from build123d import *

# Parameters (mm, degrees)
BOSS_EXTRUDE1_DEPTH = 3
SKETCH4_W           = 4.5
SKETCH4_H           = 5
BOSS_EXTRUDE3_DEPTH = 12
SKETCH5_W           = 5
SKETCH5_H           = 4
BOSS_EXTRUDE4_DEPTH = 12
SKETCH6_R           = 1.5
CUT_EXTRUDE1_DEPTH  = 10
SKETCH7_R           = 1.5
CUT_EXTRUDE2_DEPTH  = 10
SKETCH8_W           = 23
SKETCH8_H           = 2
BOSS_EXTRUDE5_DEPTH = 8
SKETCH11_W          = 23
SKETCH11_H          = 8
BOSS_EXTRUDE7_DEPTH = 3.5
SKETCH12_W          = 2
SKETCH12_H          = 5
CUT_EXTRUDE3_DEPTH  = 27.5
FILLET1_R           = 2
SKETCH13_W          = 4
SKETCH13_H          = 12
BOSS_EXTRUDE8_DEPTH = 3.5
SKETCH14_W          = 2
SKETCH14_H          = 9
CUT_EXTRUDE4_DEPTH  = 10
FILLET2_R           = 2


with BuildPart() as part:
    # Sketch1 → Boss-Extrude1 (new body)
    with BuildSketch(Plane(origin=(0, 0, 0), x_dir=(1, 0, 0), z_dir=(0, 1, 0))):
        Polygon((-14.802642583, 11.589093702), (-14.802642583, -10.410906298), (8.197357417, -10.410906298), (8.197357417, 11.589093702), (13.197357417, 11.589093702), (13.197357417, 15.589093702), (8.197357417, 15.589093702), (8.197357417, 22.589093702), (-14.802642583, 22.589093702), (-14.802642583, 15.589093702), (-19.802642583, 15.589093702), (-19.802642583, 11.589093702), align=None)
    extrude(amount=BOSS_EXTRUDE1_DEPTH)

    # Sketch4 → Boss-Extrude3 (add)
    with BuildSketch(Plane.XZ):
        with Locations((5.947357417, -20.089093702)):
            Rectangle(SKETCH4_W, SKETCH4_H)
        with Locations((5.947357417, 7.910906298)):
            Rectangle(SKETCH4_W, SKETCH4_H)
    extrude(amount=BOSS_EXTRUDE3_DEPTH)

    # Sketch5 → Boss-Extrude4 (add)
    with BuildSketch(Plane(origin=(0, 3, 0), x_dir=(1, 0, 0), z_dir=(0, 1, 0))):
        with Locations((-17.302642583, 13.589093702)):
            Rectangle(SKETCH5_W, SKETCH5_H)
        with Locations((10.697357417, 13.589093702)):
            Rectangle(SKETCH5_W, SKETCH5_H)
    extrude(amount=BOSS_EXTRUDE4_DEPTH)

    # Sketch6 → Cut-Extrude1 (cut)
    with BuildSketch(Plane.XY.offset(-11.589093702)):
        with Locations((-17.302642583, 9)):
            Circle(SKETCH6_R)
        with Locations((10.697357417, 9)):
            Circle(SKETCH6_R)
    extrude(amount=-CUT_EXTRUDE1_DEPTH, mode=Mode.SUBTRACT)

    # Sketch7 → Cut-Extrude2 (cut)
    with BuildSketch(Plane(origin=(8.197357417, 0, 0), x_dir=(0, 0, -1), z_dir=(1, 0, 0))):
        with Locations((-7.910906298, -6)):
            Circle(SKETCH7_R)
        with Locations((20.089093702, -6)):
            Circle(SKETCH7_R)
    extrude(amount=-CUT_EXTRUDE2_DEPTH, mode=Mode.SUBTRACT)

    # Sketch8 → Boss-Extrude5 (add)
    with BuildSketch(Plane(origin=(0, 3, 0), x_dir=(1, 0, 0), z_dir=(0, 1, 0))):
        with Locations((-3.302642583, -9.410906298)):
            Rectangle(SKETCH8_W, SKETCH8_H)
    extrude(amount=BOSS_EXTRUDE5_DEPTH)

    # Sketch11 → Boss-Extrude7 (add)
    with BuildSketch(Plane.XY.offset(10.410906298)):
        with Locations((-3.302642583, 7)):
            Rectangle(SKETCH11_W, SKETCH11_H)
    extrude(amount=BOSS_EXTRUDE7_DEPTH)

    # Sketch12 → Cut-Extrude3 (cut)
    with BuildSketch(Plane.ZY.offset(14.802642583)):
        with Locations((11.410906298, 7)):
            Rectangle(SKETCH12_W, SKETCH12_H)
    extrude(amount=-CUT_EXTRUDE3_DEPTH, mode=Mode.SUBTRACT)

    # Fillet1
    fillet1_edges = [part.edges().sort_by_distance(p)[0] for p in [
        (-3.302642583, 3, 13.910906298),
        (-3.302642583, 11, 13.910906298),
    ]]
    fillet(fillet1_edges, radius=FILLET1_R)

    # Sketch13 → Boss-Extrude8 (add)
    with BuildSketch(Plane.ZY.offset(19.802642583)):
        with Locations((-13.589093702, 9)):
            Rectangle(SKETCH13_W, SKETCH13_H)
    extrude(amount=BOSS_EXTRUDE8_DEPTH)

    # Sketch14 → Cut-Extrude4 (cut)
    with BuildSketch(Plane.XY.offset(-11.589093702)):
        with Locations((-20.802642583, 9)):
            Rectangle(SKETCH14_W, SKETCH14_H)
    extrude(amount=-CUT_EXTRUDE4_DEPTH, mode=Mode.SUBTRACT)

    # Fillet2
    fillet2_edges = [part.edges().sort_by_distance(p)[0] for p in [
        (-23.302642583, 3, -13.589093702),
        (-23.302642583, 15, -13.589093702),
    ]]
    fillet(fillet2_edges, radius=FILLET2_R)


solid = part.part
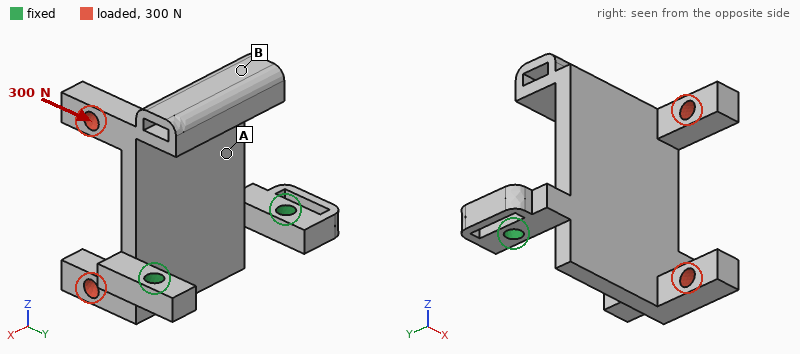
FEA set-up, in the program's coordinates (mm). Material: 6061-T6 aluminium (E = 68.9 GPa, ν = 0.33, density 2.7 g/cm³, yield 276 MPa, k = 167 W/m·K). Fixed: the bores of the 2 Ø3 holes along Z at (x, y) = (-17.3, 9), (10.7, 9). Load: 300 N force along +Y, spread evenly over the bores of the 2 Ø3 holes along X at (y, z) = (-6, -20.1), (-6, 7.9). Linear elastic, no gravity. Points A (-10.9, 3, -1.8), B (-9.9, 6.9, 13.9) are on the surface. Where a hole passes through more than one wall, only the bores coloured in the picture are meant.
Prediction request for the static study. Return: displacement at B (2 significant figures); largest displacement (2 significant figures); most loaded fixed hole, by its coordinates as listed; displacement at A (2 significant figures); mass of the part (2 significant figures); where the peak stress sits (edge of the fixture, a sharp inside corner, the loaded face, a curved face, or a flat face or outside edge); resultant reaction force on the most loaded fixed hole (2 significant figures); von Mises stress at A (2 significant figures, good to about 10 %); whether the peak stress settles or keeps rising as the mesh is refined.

0.38 mm
0.48 mm
(10.7, 9)
0.13 mm
11 g
a sharp inside corner
290 N
44 MPa
keeps rising
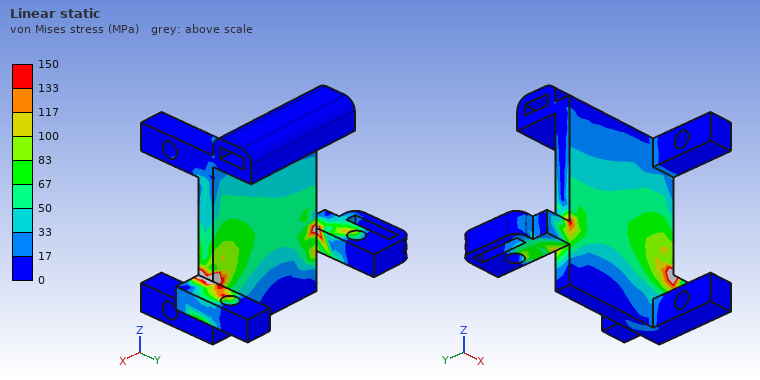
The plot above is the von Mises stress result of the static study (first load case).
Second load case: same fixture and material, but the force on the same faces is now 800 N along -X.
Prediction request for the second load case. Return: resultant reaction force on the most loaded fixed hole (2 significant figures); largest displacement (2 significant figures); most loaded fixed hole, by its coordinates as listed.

600 N
0.26 mm
(-17.3, 9)
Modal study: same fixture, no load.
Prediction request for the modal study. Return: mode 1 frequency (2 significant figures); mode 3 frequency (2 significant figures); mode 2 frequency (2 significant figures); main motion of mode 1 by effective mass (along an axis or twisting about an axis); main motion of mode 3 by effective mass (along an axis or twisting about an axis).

1400 Hz
6200 Hz
4400 Hz
along Y
along Z
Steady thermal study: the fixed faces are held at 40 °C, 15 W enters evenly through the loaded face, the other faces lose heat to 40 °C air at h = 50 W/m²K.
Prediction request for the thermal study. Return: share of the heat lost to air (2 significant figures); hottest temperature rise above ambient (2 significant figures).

27 %
47 K
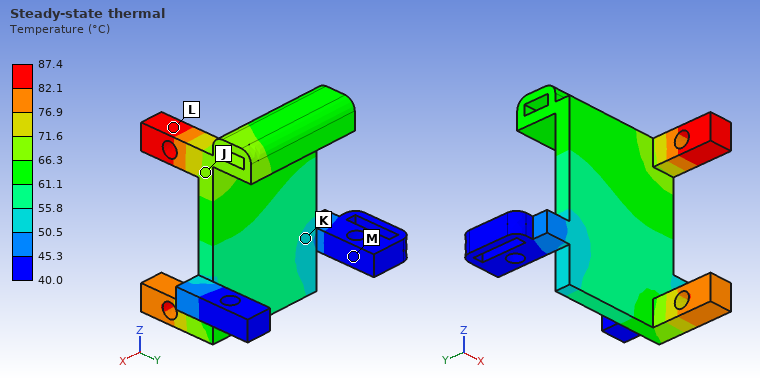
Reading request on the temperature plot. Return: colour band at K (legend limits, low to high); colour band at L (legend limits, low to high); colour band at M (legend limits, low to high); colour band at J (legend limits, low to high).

50.5 to 55.8 °C
82.1 to 87.4 °C
40.0 to 45.3 °C
66.3 to 71.6 °C
